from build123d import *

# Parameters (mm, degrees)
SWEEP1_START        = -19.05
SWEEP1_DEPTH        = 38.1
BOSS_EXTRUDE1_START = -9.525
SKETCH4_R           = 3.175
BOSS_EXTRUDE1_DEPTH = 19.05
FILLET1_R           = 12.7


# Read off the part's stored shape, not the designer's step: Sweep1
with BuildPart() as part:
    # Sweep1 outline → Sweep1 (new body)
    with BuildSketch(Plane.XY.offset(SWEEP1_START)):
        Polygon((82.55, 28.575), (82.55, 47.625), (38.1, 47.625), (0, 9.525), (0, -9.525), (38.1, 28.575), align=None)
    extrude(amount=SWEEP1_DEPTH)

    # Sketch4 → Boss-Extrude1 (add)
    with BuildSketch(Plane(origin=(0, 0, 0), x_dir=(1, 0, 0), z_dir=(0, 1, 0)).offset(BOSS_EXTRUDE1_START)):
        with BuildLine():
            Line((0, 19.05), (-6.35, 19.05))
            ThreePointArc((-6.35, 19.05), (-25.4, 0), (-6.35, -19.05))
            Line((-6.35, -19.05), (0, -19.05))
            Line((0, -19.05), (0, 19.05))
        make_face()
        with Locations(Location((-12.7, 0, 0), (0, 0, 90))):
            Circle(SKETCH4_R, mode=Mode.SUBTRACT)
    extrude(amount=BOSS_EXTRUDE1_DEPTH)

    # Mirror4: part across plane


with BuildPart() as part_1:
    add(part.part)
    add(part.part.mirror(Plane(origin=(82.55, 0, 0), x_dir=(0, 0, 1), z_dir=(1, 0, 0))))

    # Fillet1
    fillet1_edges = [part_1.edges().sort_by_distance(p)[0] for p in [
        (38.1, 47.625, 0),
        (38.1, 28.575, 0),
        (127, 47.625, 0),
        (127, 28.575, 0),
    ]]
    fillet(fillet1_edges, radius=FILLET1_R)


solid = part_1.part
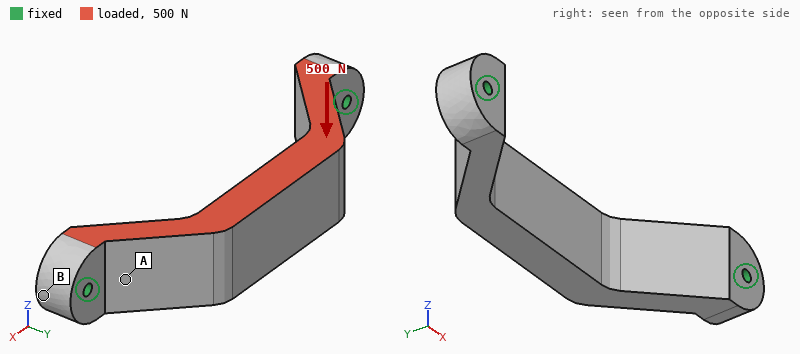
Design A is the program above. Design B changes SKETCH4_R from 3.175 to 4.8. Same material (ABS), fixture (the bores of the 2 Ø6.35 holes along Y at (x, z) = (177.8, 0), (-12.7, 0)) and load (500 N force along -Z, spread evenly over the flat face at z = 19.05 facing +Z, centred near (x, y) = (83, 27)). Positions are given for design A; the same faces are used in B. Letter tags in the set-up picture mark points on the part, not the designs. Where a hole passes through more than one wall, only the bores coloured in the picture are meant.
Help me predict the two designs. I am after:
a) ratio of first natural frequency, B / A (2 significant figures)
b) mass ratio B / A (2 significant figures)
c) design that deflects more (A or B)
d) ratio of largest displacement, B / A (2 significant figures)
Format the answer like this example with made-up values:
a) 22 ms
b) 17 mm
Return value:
a) 1.2
b) 0.99
c) A
d) 0.72
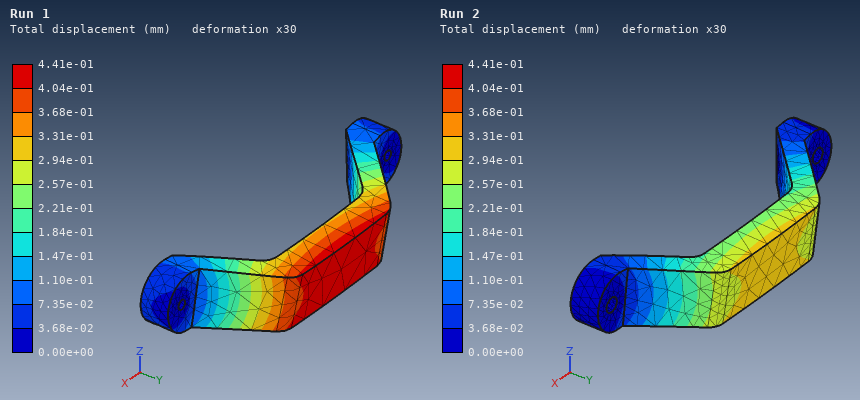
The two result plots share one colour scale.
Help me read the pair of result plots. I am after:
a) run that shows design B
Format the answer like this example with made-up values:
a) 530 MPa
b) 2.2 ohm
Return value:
a) Run 2
